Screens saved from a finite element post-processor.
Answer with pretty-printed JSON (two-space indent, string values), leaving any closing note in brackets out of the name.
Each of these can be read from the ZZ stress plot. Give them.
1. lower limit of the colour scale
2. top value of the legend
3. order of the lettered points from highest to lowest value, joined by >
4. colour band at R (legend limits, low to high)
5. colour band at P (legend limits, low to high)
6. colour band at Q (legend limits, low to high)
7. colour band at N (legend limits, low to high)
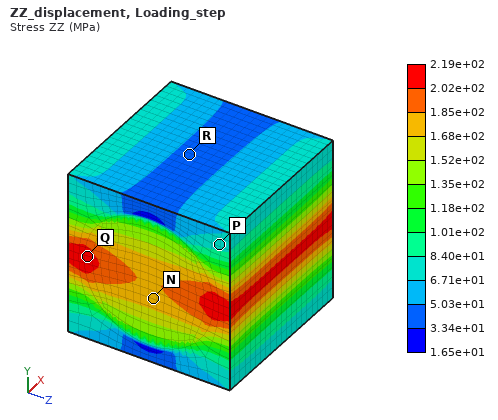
{
  "lower limit of the colour scale": "1.65e+01 MPa",
  "top value of the legend": "2.19e+02 MPa",
  "order of the lettered points from highest to lowest value, joined by >": "Q > N > P > R",
  "colour band at R": "3.34e+01 to 5.03e+01 MPa",
  "colour band at P": "6.71e+01 to 8.40e+01 MPa",
  "colour band at Q": "2.02e+02 to 2.19e+02 MPa",
  "colour band at N": "1.68e+02 to 1.85e+02 MPa"
}
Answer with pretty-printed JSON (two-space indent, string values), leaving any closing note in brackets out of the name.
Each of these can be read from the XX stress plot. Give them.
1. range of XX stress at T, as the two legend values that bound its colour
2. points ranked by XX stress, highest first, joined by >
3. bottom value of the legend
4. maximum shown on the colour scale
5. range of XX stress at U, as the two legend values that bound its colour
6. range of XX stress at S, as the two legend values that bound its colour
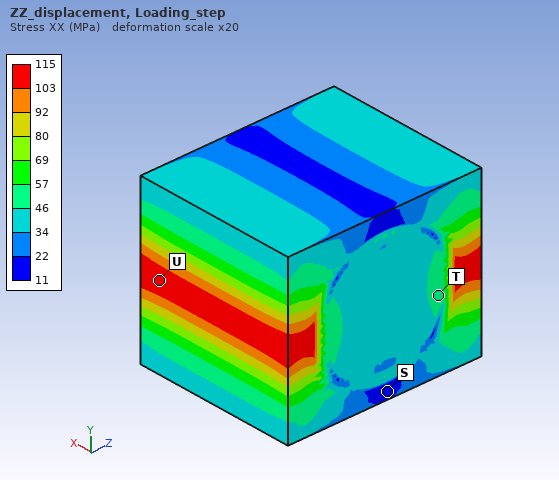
{
  "range of XX stress at T, as the two legend values that bound its colour": "46 to 57 MPa",
  "points ranked by XX stress, highest first, joined by >": "U > T > S",
  "bottom value of the legend": "11 MPa",
  "maximum shown on the colour scale": "115 MPa",
  "range of XX stress at U, as the two legend values that bound its colour": "103 to 115 MPa",
  "range of XX stress at S, as the two legend values that bound its colour": "11 to 22 MPa"
}
